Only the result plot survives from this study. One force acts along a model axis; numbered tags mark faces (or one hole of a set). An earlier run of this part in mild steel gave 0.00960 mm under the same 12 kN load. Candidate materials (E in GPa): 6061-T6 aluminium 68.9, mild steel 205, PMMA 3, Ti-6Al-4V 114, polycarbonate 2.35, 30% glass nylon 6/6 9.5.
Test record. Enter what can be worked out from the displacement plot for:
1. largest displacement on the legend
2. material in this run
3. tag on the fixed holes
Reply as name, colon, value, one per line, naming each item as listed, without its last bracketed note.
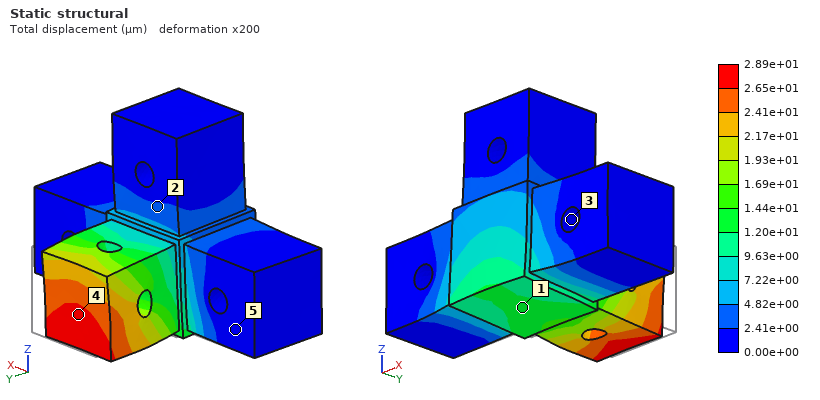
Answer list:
largest displacement on the legend: 2.89e+01 µm
material in this run: 6061-T6 aluminium
tag on the fixed holes: 3
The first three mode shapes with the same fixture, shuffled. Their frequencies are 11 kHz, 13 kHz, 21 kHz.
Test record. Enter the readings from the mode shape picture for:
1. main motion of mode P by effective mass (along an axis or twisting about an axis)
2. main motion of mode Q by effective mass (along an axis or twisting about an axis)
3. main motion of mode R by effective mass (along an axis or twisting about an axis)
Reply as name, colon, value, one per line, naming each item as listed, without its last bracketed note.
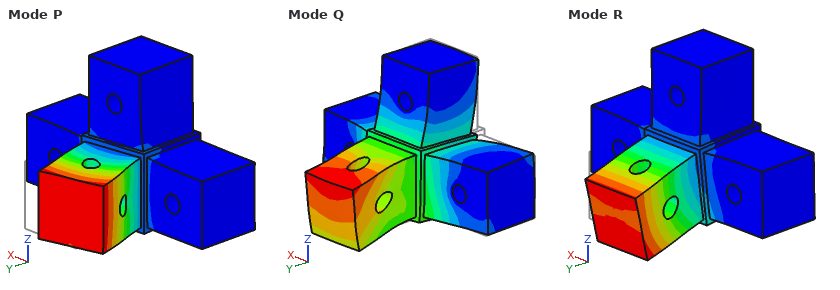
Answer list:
main motion of mode P by effective mass: along X
main motion of mode Q by effective mass: along Y
main motion of mode R by effective mass: along Z
